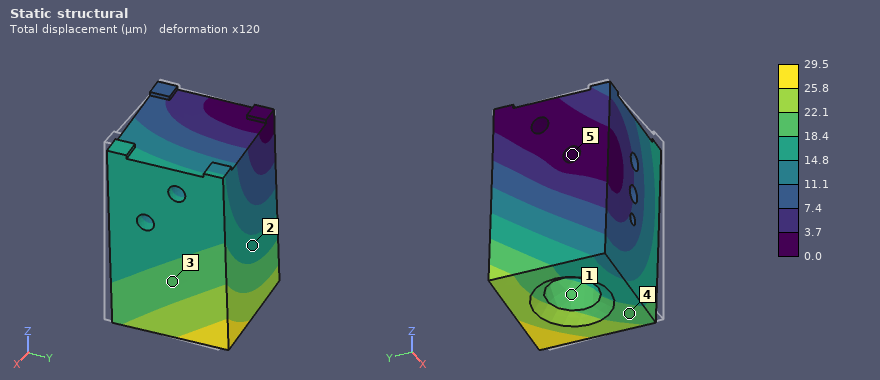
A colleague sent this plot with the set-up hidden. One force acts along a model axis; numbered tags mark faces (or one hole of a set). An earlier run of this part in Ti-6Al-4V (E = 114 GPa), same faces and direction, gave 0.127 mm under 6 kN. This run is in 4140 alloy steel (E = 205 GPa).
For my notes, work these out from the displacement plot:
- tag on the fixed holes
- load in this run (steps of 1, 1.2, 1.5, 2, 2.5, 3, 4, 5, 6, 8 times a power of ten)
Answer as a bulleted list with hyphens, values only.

- 5
- 2.5 kN
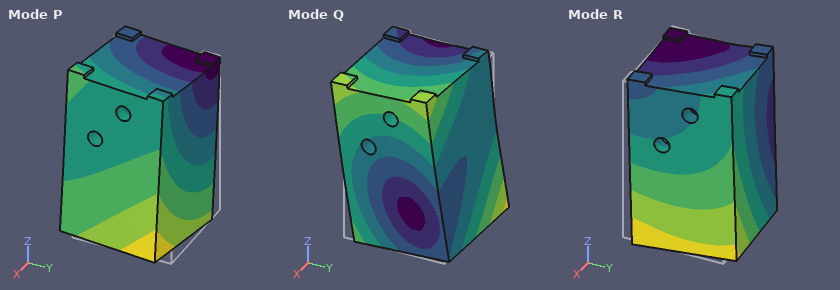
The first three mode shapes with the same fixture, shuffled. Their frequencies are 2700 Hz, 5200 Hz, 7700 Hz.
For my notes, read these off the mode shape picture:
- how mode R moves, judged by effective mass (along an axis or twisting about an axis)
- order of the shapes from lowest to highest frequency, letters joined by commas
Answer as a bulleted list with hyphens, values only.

- along Y
- P, R, Q
